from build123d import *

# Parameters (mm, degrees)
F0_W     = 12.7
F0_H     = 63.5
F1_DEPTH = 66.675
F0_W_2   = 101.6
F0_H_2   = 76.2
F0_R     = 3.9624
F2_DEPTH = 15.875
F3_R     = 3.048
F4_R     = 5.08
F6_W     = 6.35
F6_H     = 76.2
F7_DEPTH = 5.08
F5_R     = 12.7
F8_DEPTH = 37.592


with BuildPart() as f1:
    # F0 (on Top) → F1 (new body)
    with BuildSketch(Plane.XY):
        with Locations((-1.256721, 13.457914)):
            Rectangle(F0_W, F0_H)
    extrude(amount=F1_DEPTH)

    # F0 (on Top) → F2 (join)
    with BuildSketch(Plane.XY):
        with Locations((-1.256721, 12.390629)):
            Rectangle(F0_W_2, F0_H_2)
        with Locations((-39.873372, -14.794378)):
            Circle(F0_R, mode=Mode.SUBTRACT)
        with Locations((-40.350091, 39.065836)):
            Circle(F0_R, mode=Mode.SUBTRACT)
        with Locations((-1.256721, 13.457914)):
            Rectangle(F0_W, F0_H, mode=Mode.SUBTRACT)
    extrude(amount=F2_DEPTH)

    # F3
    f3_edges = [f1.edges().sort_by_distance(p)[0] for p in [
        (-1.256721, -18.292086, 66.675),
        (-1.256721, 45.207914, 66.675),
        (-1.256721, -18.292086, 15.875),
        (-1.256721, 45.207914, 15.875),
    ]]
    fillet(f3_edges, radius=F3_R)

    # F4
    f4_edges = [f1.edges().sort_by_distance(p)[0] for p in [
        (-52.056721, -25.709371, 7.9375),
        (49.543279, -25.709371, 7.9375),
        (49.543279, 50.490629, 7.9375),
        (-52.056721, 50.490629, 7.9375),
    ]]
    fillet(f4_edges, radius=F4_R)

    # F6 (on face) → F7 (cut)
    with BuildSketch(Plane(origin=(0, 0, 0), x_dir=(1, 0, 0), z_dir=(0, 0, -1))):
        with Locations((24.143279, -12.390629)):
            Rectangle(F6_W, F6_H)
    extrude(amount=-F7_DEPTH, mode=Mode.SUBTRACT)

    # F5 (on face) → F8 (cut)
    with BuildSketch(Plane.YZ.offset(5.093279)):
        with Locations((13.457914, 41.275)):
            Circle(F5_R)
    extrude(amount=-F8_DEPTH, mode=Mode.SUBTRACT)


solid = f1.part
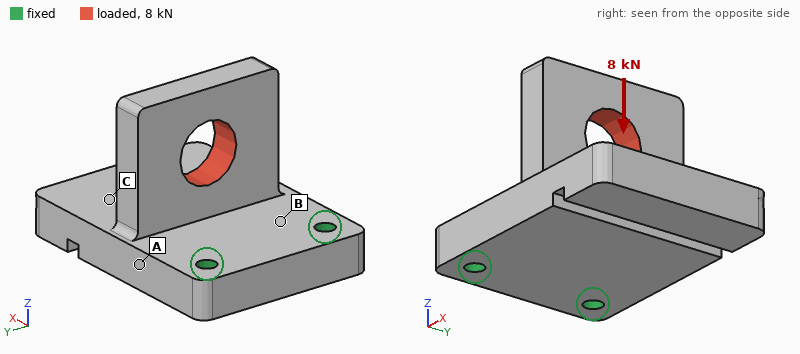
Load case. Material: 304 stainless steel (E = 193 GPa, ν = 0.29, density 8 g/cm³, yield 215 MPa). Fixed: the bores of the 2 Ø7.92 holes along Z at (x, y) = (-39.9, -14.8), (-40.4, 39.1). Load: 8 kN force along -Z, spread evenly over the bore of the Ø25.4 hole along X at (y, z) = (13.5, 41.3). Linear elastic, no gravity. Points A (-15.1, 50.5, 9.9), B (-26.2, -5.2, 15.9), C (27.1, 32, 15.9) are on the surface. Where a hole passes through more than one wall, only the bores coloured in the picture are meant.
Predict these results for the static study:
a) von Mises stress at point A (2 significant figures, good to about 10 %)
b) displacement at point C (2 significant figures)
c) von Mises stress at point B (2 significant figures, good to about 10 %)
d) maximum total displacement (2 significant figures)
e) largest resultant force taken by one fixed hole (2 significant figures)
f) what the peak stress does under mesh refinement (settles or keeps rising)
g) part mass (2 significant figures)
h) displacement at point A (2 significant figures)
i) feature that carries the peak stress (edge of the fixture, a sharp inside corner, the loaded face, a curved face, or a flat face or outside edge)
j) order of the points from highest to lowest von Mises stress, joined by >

33 MPa
0.087 mm
56 MPa
0.12 mm
4.1 kN
keeps rising
1.2 kg
0.022 mm
edge of the fixture
B > A > C
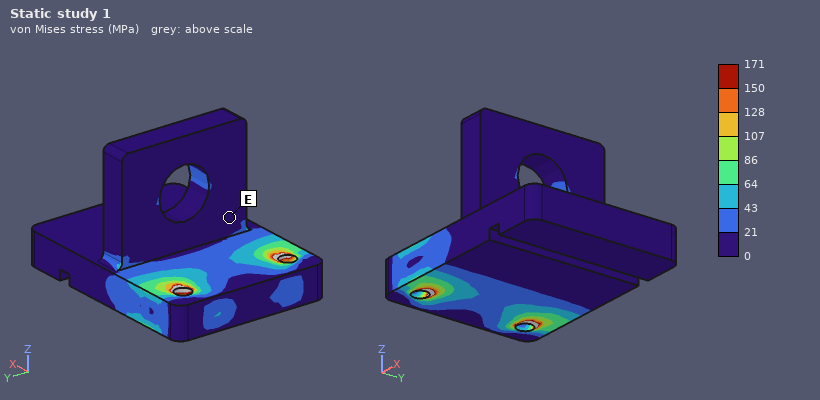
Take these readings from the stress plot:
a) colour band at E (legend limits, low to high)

0 to 21 MPa
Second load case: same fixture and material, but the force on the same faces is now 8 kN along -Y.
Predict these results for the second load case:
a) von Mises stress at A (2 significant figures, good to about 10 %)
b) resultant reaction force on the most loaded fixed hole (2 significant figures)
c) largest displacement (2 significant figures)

52 MPa
8.0 kN
62 µm
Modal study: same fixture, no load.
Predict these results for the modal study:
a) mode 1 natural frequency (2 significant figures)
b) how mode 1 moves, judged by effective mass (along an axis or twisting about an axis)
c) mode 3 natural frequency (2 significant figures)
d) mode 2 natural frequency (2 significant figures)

1200 Hz
along Z
3300 Hz
3100 Hz
